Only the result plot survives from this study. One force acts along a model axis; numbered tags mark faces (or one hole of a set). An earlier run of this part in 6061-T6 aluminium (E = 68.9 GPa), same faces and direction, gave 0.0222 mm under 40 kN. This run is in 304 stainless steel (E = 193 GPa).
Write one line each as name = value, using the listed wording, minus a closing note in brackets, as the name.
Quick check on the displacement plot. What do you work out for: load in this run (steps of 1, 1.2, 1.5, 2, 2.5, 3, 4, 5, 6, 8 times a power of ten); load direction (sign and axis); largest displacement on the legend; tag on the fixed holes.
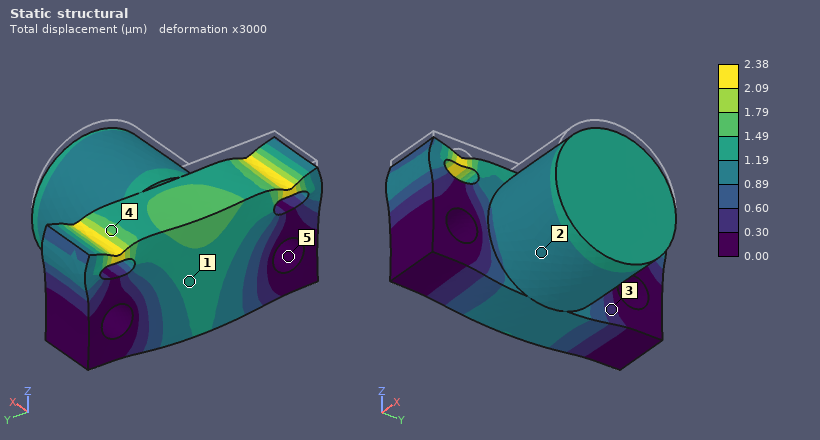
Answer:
load in this run = 12 kN
load direction = -Z
largest displacement on the legend = 2.38 µm
tag on the fixed holes = 5
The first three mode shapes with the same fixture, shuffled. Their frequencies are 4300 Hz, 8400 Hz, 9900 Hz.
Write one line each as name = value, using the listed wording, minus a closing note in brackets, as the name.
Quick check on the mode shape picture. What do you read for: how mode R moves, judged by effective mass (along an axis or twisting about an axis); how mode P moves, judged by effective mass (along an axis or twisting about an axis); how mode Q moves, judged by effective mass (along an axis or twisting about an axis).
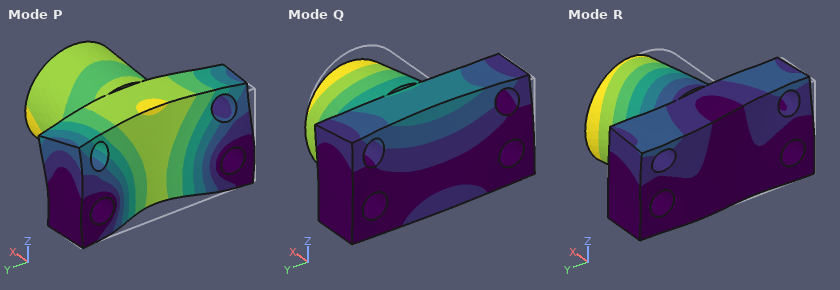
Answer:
how mode R moves, judged by effective mass = along Y
how mode P moves, judged by effective mass = along X
how mode Q moves, judged by effective mass = along Z
